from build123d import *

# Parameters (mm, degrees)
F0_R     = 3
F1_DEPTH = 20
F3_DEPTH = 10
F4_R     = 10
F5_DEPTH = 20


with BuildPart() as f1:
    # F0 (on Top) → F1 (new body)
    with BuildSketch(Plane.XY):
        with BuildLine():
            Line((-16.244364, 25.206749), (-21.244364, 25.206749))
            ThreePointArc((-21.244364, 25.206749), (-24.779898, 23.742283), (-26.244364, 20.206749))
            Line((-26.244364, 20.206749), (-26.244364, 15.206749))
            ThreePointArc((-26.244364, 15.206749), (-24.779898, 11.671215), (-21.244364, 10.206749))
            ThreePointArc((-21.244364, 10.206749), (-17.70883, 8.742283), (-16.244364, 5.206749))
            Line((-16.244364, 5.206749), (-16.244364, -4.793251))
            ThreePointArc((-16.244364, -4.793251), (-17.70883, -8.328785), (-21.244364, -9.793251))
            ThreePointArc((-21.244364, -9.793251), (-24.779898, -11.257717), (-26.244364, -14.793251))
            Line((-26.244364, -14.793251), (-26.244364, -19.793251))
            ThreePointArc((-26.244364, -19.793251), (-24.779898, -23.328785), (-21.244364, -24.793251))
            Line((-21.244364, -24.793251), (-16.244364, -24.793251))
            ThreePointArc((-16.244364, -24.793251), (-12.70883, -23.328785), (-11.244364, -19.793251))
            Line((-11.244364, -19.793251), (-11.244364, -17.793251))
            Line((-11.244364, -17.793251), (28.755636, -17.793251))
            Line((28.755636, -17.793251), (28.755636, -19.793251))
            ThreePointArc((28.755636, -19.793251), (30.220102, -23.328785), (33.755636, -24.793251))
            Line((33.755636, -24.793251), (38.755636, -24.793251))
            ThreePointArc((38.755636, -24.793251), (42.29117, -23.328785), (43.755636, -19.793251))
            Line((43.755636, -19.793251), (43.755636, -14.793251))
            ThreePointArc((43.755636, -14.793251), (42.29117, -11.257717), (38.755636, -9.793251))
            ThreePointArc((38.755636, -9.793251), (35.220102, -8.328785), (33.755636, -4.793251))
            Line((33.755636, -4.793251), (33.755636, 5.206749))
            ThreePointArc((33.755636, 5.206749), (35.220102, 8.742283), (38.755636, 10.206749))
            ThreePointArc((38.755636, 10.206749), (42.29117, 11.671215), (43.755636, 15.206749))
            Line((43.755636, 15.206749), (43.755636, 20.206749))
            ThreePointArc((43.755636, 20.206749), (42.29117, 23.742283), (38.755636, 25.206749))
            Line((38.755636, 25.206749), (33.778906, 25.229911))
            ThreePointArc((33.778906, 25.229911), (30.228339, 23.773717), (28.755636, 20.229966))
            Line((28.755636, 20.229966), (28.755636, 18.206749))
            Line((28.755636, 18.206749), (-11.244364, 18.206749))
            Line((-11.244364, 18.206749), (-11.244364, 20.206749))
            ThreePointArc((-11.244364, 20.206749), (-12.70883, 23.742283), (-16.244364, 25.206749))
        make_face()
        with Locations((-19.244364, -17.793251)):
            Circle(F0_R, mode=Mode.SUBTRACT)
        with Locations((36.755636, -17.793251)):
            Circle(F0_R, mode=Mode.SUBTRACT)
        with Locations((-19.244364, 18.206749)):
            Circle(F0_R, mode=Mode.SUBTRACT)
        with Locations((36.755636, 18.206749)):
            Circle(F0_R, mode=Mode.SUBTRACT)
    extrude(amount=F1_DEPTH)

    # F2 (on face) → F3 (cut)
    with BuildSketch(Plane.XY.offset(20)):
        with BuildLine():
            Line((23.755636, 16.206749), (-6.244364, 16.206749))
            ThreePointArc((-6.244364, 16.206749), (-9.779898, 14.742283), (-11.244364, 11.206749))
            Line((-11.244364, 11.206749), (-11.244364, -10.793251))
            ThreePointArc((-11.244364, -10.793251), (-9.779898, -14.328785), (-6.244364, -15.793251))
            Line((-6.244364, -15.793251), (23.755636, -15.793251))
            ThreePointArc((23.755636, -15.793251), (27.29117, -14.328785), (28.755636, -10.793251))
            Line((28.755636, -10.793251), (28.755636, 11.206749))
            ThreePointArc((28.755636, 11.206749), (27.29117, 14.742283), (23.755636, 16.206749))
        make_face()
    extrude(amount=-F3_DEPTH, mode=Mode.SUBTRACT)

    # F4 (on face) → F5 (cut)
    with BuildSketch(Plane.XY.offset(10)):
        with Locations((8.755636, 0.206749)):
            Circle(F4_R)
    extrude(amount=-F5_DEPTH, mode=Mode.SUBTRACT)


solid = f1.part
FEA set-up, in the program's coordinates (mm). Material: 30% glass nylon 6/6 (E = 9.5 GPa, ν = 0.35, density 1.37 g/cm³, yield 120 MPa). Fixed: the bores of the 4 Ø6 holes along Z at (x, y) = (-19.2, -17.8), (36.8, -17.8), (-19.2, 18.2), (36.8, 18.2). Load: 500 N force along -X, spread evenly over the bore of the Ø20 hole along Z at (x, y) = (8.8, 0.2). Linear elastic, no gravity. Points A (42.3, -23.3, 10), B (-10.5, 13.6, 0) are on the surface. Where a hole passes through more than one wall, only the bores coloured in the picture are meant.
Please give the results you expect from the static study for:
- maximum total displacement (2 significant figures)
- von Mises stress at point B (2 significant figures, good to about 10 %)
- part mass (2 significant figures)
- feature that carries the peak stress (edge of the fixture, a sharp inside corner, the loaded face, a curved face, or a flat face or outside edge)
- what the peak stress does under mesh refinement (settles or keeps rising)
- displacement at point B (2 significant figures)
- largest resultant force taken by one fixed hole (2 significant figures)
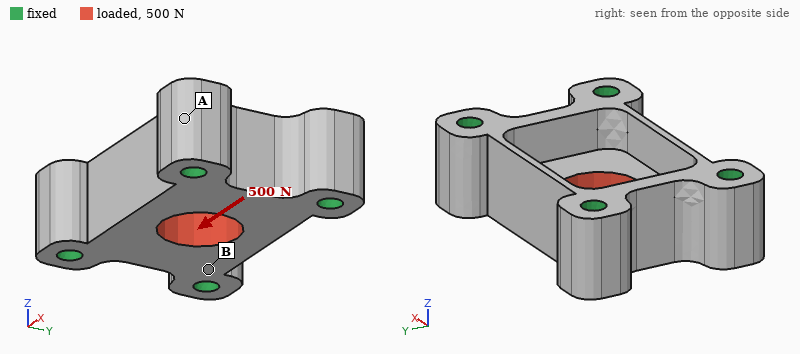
2.6 µm
0.87 MPa
44 g
edge of the fixture
keeps rising
0.97 µm
140 N
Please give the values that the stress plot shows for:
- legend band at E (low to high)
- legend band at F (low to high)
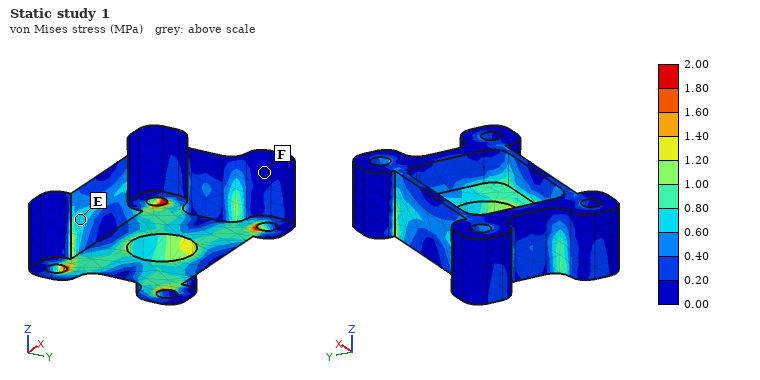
0.60 to 0.80 MPa
0.00 to 0.20 MPa
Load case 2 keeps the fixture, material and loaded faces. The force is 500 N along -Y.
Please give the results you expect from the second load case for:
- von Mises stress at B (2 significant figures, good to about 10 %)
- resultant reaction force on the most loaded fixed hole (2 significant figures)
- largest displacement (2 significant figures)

0.98 MPa
160 N
6.5 µm
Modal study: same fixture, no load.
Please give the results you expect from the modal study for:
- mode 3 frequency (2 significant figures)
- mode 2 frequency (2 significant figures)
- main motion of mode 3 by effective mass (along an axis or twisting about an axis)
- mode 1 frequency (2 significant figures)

11 kHz
9300 Hz
along Z
9200 Hz
